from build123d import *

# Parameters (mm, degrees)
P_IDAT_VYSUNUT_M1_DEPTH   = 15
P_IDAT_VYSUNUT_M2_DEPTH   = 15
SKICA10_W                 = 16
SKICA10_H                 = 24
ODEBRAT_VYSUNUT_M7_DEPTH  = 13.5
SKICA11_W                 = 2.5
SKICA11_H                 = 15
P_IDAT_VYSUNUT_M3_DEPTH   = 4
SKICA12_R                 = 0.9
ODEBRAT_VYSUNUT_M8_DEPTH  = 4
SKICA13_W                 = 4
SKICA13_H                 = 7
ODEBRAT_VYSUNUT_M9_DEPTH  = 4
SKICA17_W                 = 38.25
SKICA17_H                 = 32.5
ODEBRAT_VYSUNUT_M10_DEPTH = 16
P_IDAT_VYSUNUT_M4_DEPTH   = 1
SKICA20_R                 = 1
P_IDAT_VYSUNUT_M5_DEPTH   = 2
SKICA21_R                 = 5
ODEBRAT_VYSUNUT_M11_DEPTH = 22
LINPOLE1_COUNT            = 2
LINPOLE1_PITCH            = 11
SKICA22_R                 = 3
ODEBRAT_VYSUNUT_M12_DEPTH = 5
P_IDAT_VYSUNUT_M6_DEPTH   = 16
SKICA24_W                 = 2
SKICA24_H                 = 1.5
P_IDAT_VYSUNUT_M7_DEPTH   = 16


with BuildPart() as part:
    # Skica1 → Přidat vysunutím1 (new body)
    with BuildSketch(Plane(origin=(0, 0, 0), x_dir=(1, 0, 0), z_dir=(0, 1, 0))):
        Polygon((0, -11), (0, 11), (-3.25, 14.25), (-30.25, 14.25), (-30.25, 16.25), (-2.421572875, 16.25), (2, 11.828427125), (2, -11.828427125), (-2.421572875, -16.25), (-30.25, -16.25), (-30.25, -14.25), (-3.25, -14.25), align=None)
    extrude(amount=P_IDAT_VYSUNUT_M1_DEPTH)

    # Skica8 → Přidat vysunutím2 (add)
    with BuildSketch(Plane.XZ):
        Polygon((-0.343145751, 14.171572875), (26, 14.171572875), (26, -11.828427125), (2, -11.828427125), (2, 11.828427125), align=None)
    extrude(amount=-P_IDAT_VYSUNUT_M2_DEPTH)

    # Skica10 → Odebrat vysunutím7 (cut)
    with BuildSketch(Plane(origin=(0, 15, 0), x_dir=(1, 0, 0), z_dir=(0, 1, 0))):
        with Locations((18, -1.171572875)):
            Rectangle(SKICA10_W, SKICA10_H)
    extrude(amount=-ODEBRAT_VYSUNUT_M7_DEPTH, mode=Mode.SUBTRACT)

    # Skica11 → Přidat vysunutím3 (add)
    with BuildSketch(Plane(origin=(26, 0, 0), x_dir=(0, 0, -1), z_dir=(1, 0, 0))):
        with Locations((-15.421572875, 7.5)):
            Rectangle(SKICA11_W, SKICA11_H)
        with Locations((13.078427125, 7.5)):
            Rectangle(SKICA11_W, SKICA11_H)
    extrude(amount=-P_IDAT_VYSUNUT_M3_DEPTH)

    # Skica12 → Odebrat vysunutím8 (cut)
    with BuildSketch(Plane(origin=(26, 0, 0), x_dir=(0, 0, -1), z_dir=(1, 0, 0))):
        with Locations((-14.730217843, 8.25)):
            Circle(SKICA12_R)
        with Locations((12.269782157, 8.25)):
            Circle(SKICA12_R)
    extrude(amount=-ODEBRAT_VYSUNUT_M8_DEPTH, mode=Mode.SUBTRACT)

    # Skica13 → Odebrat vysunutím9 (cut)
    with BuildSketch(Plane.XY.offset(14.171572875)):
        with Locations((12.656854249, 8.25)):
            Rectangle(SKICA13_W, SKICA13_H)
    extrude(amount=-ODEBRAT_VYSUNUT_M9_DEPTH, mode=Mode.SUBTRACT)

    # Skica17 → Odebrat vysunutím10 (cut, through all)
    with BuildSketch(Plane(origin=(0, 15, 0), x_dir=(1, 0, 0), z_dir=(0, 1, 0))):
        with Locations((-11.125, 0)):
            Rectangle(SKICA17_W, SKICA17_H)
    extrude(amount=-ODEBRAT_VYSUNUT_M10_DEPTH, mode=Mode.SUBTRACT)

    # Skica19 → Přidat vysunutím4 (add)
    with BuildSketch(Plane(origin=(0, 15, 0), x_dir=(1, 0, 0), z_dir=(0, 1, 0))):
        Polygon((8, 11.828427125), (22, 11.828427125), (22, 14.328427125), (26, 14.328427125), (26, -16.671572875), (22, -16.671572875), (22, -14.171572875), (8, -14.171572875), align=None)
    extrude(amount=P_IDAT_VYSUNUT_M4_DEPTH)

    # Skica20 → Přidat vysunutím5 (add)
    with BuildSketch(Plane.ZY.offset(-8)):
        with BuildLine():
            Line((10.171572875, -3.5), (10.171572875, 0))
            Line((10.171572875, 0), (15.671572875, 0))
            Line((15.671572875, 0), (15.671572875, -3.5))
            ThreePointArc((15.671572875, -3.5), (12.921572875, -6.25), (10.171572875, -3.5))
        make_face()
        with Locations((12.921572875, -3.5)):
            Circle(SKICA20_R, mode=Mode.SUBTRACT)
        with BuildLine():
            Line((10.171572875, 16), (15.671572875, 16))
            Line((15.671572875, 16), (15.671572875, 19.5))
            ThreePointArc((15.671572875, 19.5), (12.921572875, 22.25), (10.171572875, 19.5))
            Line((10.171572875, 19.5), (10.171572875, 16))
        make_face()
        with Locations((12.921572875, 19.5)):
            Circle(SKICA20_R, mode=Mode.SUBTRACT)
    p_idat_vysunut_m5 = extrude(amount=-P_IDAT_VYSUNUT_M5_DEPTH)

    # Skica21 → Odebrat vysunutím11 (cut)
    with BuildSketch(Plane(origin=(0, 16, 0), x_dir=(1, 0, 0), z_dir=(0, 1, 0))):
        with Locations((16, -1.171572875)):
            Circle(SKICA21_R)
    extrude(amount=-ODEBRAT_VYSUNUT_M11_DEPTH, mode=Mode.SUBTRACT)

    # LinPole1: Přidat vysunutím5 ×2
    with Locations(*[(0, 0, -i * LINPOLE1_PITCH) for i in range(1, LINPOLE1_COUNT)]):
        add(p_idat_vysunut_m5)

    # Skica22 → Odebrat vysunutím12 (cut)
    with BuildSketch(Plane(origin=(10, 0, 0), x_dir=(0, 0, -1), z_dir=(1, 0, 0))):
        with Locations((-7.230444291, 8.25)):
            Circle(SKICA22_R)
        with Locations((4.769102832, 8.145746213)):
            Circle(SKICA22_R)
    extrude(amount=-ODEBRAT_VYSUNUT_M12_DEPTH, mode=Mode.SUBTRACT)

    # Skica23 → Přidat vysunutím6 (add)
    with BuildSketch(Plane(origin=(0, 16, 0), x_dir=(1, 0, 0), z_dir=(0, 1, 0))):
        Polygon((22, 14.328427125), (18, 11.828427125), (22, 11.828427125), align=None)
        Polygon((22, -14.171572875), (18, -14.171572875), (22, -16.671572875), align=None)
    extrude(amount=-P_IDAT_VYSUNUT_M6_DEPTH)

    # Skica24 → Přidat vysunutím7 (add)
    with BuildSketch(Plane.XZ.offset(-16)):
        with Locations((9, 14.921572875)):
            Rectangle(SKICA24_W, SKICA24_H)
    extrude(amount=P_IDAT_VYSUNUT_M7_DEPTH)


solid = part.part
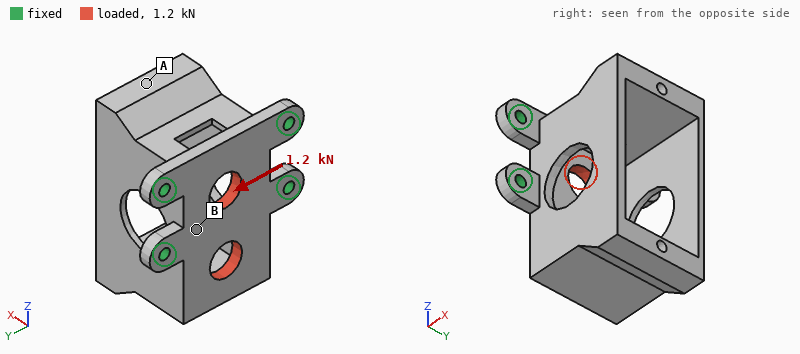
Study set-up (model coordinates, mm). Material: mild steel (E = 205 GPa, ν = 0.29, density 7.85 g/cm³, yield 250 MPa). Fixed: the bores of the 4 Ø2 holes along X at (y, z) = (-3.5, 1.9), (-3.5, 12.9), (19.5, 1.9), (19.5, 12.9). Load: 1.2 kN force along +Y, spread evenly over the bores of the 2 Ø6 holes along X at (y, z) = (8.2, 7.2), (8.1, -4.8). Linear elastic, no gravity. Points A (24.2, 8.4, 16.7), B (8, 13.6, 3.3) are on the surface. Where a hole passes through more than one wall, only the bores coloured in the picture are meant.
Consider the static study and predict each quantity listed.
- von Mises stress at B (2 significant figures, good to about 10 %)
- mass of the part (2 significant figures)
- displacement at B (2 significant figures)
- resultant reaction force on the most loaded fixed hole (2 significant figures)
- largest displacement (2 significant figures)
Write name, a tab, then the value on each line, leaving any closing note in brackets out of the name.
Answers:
von Mises stress at B	23 MPa
mass of the part	21 g
displacement at B	0.96 µm
resultant reaction force on the most loaded fixed hole	460 N
largest displacement	5.4 µm
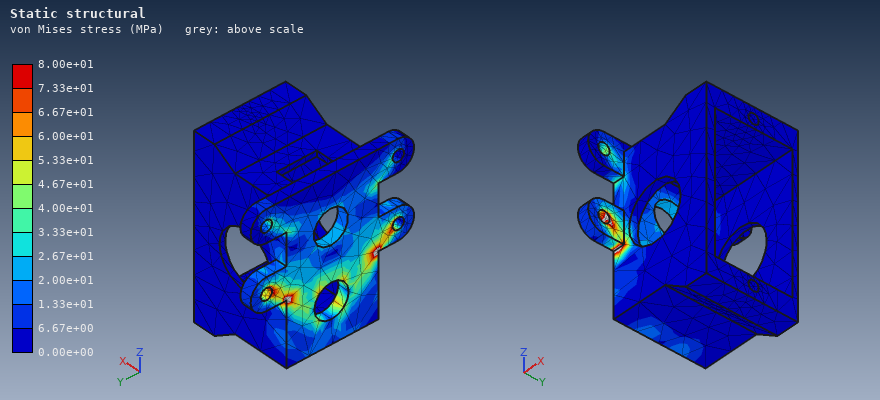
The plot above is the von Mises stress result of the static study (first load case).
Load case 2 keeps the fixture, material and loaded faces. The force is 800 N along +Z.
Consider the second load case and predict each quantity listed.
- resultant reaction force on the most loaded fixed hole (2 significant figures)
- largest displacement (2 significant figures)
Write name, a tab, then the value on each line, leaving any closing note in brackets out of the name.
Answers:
resultant reaction force on the most loaded fixed hole	240 N
largest displacement	2.7 µm
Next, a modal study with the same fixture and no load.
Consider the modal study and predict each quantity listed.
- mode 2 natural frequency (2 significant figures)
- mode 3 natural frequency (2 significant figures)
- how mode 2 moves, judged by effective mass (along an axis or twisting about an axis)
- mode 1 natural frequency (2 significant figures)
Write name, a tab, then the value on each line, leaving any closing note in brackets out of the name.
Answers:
mode 2 natural frequency	5800 Hz
mode 3 natural frequency	9900 Hz
how mode 2 moves, judged by effective mass	along Y
mode 1 natural frequency	5200 Hz
